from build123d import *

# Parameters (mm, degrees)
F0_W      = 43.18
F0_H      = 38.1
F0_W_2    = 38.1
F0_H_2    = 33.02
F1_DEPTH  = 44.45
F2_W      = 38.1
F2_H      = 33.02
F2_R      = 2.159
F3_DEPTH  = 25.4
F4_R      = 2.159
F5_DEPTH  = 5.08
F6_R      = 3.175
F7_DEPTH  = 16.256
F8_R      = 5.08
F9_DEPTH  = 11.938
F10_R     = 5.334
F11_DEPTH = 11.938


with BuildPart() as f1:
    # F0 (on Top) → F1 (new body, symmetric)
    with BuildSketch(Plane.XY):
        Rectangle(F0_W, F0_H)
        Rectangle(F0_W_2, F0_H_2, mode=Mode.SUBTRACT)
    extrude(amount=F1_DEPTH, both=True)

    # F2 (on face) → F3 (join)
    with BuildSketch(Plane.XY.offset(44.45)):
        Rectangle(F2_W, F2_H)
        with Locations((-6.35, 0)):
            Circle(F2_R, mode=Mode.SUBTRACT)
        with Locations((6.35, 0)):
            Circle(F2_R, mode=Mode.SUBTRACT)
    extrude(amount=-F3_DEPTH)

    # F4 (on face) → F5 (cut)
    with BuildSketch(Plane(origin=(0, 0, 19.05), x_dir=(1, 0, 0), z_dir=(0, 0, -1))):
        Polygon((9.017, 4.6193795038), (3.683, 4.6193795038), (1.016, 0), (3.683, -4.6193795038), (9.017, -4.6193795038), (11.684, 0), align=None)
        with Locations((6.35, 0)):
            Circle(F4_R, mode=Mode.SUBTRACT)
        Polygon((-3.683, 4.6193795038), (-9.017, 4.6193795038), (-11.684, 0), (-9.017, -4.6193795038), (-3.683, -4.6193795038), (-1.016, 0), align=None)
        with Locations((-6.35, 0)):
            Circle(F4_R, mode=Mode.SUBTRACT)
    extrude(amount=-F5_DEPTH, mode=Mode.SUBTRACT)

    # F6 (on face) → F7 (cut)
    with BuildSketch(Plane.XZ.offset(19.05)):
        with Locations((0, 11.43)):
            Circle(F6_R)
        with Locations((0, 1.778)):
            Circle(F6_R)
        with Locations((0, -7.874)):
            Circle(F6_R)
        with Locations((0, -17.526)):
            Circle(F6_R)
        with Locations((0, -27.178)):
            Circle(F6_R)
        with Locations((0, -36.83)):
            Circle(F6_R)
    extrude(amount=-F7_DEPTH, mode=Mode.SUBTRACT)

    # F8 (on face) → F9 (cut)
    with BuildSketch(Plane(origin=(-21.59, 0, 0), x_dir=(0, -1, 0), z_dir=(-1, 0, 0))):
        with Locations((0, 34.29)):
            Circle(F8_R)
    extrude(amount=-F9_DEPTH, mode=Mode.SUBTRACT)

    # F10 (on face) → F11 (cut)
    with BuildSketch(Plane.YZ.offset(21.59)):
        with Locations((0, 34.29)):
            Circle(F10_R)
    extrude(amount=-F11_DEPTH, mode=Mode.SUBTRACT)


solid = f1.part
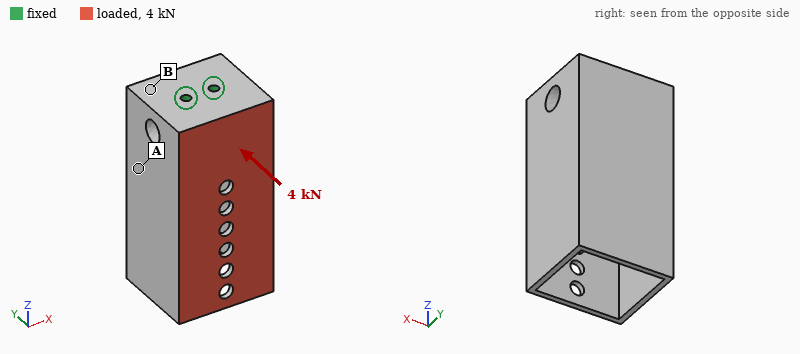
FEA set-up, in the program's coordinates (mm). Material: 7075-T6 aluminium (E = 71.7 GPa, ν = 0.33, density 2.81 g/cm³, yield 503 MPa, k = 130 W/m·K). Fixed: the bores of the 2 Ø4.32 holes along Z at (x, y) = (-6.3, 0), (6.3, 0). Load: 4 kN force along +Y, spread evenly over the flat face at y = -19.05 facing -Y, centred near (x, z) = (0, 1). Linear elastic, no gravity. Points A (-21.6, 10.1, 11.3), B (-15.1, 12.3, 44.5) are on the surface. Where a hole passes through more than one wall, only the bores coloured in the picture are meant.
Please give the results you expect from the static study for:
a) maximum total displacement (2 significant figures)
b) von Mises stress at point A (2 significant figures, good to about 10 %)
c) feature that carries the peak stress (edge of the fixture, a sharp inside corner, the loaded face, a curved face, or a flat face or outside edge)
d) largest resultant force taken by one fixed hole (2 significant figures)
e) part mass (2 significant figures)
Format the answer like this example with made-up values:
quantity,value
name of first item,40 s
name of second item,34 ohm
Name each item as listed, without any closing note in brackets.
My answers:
quantity,value
maximum total displacement,0.28 mm
von Mises stress at point A,34 MPa
feature that carries the peak stress,the loaded face
largest resultant force taken by one fixed hole,2.0 kN
part mass,180 g
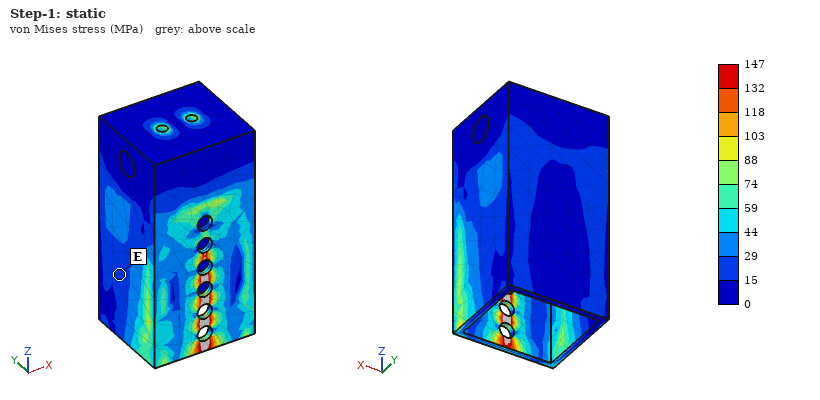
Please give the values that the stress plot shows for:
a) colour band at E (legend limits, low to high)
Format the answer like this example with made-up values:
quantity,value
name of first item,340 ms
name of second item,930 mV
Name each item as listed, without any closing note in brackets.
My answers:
quantity,value
colour band at E,15 to 29 MPa
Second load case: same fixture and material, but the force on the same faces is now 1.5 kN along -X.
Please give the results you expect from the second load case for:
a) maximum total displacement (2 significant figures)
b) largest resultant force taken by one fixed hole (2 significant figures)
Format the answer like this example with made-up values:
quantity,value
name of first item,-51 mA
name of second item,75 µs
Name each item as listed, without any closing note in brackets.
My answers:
quantity,value
maximum total displacement,59 µm
largest resultant force taken by one fixed hole,2.5 kN
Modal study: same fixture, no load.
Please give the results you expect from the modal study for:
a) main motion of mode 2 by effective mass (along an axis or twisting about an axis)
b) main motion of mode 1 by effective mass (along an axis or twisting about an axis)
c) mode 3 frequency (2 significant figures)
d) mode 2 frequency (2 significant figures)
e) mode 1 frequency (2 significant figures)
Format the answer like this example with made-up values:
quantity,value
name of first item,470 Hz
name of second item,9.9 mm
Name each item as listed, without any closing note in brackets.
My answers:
quantity,value
main motion of mode 2 by effective mass,along X
main motion of mode 1 by effective mass,along Y
mode 3 frequency,4300 Hz
mode 2 frequency,3900 Hz
mode 1 frequency,3600 Hz
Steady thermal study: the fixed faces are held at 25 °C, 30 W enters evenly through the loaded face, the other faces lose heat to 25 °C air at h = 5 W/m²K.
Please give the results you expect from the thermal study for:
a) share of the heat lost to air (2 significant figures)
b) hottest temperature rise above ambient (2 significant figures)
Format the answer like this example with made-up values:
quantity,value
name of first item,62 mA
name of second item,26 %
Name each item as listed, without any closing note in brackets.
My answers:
quantity,value
share of the heat lost to air,3.7 %
hottest temperature rise above ambient,24 K
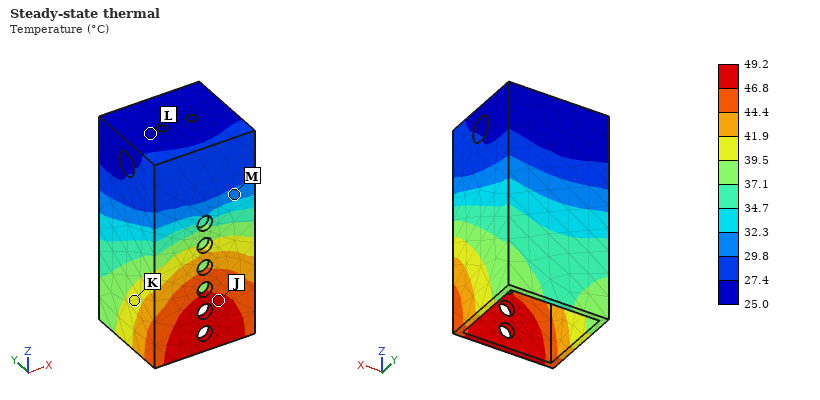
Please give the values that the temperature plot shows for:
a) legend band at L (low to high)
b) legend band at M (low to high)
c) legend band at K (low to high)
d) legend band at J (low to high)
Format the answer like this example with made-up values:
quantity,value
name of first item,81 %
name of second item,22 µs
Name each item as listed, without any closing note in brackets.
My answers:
quantity,value
legend band at L,25.0 to 27.4 °C
legend band at M,29.8 to 32.3 °C
legend band at K,39.5 to 41.9 °C
legend band at J,46.8 to 49.2 °C
